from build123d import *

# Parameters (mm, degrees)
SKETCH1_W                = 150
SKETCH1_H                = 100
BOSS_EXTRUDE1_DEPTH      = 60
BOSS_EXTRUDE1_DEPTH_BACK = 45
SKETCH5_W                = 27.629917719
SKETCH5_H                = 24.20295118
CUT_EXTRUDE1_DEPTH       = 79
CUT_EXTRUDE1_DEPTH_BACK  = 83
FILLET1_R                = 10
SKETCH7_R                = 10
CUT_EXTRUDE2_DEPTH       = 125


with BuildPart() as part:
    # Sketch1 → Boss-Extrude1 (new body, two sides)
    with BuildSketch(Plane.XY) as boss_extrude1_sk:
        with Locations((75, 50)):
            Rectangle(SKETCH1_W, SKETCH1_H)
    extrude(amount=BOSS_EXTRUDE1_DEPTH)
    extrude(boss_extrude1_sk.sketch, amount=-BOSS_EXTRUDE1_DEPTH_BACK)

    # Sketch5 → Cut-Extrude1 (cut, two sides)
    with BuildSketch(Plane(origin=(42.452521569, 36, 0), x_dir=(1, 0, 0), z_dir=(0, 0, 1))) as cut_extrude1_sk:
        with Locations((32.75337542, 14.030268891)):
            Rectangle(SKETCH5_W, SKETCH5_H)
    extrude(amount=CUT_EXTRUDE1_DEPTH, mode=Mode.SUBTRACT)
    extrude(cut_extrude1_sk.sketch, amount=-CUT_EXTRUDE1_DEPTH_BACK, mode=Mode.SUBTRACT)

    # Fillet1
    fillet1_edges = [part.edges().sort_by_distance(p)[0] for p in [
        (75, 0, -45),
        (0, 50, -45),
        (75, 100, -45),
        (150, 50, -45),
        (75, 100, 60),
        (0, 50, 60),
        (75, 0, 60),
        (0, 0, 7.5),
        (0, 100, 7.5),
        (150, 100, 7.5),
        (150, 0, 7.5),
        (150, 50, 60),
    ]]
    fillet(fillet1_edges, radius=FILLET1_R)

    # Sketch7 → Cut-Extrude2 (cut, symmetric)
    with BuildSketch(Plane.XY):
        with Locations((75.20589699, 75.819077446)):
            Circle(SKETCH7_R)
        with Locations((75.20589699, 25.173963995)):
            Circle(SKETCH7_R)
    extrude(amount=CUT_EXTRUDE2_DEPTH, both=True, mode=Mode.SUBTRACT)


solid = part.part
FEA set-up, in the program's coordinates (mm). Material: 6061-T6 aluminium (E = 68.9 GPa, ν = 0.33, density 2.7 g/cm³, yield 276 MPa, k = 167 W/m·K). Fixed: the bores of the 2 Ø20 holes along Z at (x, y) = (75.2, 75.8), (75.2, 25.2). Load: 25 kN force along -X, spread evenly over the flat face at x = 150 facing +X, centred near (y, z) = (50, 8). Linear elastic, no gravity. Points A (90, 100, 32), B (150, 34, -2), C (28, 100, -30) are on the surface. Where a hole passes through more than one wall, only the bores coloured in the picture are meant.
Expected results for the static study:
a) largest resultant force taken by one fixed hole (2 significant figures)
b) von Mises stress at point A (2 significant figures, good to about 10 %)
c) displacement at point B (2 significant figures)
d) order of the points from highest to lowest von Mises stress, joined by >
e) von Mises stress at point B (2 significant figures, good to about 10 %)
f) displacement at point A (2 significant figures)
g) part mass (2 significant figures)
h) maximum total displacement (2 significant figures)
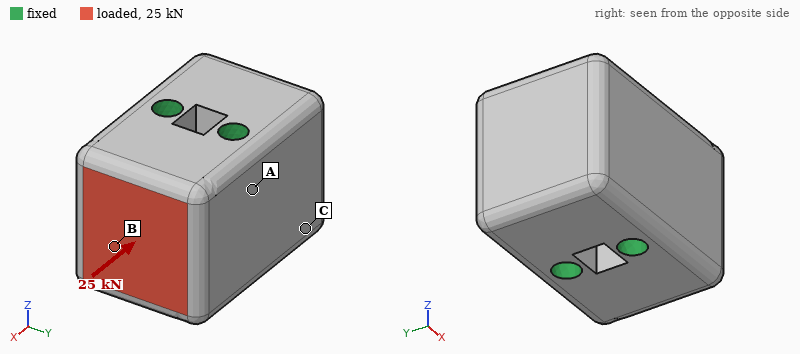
13 kN
1.3 MPa
3.3 µm
B > A > C
2.2 MPa
0.86 µm
3.8 kg
3.4 µm
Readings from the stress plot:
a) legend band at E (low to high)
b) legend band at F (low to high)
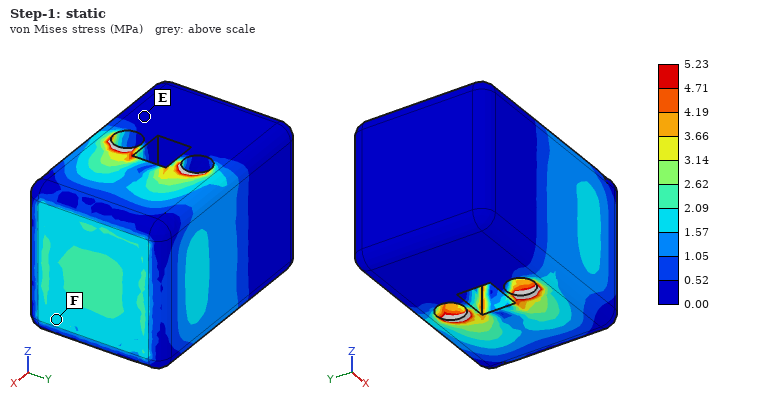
0.00 to 0.52 MPa
1.57 to 2.09 MPa
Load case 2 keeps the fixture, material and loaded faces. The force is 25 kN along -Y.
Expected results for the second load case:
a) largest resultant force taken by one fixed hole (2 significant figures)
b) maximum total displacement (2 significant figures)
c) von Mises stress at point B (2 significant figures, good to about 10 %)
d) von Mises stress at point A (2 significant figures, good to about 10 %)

28 kN
16 µm
6.5 MPa
6.7 MPa
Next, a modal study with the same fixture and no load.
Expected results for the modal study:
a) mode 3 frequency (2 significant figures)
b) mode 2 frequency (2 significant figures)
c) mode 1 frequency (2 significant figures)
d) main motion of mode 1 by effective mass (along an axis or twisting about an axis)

8300 Hz
8100 Hz
7200 Hz
twisting about Z
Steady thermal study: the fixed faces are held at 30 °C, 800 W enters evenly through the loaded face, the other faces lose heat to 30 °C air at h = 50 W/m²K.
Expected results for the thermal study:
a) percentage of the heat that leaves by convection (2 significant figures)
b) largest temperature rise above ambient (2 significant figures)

3.4 %
39 K
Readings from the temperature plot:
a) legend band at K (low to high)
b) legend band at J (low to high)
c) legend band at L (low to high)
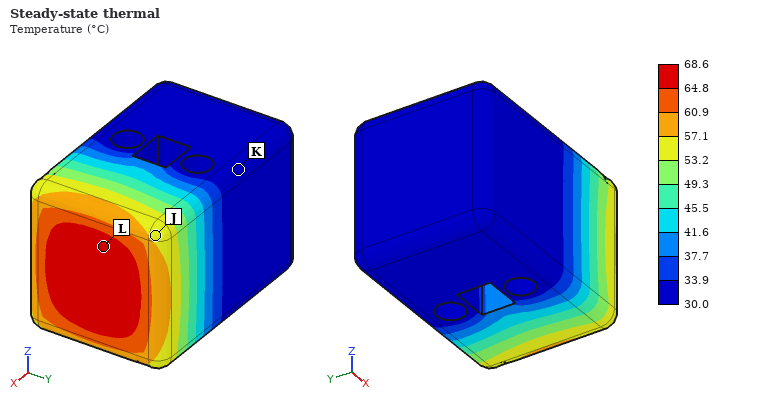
30.0 to 33.9 °C
53.2 to 57.1 °C
64.8 to 68.6 °C
